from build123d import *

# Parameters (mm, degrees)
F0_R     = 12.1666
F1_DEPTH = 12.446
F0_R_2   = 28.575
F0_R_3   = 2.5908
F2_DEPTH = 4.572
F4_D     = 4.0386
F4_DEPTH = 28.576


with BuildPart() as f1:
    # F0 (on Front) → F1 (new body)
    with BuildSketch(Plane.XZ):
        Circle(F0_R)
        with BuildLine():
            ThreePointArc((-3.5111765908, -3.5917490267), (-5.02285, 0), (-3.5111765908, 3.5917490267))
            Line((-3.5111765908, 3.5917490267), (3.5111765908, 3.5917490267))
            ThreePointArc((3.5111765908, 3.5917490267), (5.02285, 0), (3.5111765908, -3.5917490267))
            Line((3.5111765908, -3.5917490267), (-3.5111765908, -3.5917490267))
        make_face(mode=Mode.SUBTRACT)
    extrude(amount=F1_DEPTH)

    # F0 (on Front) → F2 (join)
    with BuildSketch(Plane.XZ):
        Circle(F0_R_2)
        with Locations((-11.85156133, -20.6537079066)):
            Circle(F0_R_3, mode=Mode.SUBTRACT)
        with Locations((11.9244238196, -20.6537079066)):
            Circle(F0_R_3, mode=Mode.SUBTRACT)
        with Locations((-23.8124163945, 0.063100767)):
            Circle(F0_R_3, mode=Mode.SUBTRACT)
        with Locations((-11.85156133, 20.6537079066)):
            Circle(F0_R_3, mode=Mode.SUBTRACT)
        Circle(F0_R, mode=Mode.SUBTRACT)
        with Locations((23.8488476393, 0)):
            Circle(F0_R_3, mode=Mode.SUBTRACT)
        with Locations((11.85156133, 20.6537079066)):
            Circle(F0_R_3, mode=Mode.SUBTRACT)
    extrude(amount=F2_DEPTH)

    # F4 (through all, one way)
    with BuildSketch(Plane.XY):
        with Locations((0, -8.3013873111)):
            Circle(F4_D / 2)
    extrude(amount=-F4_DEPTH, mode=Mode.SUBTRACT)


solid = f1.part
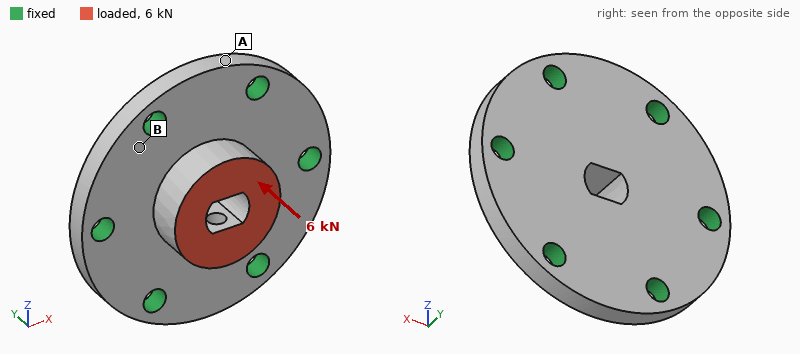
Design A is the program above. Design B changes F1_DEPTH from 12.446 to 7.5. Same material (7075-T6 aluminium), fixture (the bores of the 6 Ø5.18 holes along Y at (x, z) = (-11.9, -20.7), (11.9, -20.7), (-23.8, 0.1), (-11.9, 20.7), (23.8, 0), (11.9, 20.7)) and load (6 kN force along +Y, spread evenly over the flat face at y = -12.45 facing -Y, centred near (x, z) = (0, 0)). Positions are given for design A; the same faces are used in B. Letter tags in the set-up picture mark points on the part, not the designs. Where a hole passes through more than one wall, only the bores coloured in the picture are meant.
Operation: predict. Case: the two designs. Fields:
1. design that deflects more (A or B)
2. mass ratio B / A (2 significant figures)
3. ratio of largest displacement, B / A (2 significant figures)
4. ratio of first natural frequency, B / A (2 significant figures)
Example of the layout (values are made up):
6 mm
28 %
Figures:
B
0.86
1.5
1.1
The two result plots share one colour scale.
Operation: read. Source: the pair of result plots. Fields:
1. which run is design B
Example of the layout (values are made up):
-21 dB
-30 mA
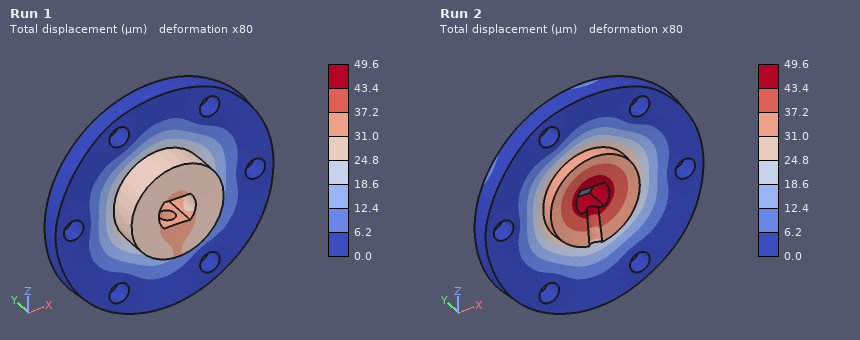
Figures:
Run 2
